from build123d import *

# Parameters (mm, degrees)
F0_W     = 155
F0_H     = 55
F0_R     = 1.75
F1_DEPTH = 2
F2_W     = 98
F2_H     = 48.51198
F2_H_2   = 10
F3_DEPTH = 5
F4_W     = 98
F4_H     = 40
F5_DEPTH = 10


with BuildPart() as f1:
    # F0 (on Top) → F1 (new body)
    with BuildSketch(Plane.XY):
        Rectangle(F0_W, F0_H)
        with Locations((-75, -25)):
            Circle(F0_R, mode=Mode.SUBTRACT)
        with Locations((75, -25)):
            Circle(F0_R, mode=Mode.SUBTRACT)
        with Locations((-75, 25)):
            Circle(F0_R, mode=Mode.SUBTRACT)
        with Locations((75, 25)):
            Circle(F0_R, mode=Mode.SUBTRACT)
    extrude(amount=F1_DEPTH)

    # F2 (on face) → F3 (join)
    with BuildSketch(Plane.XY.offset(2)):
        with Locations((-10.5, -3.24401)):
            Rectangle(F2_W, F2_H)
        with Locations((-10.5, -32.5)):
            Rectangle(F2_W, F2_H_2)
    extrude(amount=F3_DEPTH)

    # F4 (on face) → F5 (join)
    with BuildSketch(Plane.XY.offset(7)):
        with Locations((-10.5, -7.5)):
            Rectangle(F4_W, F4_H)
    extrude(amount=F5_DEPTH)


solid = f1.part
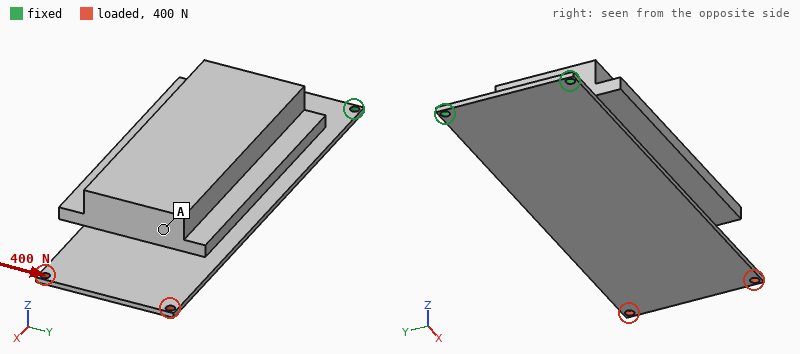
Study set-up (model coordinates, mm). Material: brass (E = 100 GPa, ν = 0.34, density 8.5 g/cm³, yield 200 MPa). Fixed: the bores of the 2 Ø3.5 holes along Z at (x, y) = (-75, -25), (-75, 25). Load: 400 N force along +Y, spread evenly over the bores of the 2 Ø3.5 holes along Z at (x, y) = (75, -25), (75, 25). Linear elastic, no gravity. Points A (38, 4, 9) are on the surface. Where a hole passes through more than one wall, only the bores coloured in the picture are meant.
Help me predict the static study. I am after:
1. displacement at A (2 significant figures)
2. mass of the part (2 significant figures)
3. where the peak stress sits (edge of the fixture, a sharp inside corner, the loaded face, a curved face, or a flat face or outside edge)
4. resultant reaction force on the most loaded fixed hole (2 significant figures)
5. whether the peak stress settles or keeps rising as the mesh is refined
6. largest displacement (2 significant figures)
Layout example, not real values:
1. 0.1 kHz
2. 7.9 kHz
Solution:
1. 0.071 mm
2. 720 g
3. edge of the fixture
4. 1.2 kN
5. keeps rising
6. 0.12 mm
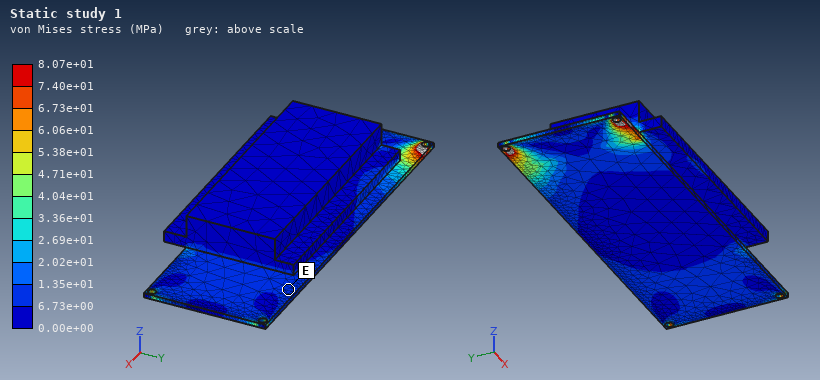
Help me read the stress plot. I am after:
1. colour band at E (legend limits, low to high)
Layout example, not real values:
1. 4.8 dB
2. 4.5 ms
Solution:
1. 6.73e+00 to 1.35e+01 MPa
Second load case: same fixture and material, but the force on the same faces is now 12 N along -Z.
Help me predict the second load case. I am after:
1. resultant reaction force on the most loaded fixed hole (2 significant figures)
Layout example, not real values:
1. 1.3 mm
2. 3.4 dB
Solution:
1. 8.4 N
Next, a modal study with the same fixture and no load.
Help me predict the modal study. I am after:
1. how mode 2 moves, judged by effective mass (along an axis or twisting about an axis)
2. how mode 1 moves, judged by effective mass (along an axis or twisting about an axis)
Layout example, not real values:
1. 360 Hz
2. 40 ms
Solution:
1. along Y
2. along Z
